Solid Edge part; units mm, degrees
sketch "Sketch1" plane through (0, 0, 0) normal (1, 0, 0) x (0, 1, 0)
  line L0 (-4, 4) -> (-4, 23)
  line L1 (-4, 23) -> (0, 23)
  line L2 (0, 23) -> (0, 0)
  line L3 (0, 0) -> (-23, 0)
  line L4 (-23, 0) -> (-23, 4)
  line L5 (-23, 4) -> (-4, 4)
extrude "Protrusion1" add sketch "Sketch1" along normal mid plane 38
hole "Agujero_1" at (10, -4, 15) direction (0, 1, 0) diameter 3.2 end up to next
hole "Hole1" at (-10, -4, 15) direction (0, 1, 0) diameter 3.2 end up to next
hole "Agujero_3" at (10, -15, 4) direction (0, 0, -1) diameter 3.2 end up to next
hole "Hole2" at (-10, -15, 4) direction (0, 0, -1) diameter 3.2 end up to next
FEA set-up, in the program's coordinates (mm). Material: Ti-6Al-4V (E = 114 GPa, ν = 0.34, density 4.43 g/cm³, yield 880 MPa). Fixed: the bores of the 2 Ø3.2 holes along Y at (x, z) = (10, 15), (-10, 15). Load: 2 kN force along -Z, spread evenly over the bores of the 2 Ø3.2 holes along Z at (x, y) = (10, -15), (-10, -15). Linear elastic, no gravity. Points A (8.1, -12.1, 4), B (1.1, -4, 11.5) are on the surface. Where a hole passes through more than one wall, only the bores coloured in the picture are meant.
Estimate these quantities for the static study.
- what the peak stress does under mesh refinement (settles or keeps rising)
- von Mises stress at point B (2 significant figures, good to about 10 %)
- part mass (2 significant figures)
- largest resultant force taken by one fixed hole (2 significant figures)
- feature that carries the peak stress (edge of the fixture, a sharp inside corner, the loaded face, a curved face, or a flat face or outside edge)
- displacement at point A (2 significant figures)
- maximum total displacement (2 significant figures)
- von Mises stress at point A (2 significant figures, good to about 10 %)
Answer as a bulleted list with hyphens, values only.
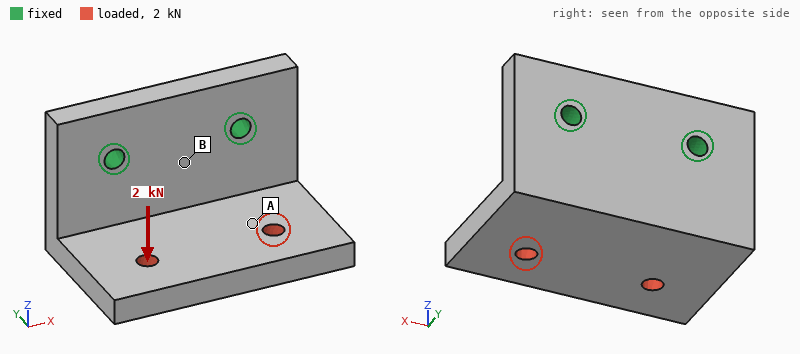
- keeps rising
- 190 MPa
- 28 g
- 1.0 kN
- edge of the fixture
- 0.19 mm
- 0.41 mm
- 65 MPa
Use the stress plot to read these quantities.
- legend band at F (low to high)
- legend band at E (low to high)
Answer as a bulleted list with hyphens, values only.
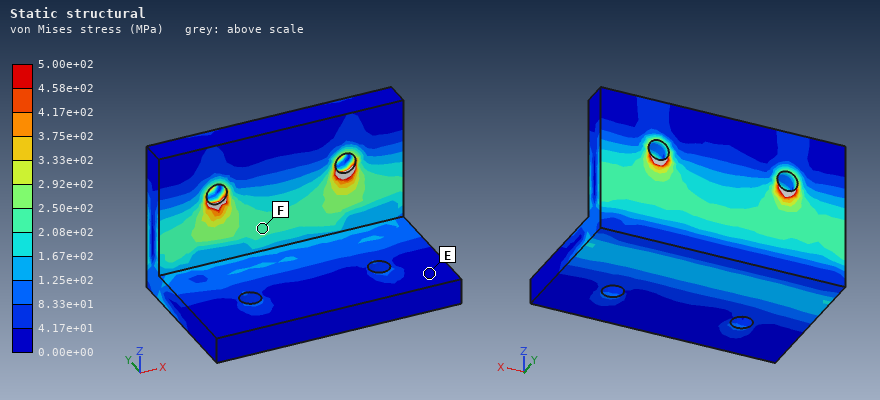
- 2.08e+02 to 2.50e+02 MPa
- 0.00e+00 to 4.17e+01 MPa
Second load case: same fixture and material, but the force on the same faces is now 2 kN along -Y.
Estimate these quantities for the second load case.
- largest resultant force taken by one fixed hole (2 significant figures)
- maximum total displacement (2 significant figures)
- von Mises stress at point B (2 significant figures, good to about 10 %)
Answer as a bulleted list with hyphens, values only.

- 1.0 kN
- 0.19 mm
- 120 MPa
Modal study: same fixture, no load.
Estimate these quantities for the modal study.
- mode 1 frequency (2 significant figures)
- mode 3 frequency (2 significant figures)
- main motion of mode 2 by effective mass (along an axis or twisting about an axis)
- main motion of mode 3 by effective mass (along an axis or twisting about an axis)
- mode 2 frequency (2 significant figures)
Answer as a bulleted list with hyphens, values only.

- 3700 Hz
- 11 kHz
- along X
- along Y
- 6400 Hz
